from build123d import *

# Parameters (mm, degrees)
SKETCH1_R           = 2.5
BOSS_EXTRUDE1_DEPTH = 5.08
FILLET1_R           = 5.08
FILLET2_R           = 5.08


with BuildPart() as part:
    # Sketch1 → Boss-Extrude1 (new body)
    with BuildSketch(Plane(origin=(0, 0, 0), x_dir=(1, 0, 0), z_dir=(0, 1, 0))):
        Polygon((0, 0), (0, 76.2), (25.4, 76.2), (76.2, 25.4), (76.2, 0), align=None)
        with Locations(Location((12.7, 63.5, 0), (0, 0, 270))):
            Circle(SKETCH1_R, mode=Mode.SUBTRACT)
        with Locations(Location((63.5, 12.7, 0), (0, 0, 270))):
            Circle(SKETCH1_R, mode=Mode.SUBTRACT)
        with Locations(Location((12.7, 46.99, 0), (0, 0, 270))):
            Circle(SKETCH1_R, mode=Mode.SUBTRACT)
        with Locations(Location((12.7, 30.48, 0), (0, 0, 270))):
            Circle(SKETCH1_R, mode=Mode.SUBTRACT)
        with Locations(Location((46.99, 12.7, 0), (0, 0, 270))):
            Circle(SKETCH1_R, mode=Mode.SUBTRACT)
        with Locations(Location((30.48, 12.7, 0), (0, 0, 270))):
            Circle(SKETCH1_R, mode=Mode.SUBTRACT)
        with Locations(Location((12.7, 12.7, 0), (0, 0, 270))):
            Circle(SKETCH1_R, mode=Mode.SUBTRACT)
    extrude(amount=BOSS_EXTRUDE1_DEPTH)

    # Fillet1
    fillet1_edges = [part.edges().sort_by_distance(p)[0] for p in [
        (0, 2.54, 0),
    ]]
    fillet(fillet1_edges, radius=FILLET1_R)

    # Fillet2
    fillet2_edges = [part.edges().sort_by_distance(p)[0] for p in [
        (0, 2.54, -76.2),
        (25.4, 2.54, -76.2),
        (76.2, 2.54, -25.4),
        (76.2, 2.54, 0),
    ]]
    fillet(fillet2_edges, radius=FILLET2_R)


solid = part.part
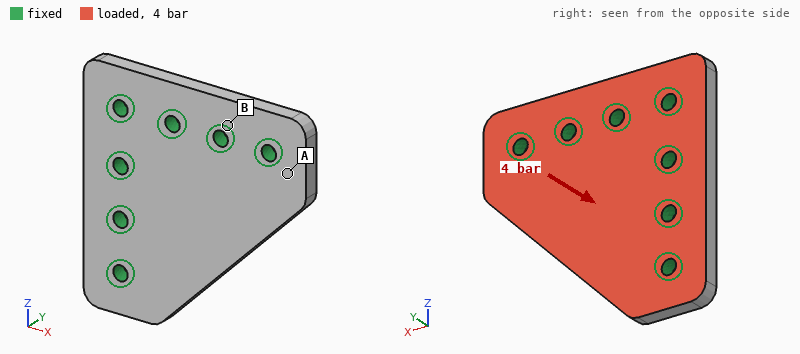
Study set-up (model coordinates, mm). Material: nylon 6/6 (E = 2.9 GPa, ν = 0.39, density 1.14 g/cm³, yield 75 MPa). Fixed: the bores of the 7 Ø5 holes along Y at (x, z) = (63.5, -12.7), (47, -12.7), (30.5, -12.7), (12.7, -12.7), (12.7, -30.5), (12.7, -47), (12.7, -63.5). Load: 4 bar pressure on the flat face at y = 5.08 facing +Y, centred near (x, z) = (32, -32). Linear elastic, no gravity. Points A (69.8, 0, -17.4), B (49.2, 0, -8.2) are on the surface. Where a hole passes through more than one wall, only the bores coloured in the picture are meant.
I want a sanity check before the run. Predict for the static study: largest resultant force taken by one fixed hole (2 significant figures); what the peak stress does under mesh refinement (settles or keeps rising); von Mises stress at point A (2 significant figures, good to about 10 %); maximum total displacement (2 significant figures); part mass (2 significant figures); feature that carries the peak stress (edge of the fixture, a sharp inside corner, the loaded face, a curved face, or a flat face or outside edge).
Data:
330 N
keeps rising
14 MPa
0.92 mm
25 g
edge of the fixture
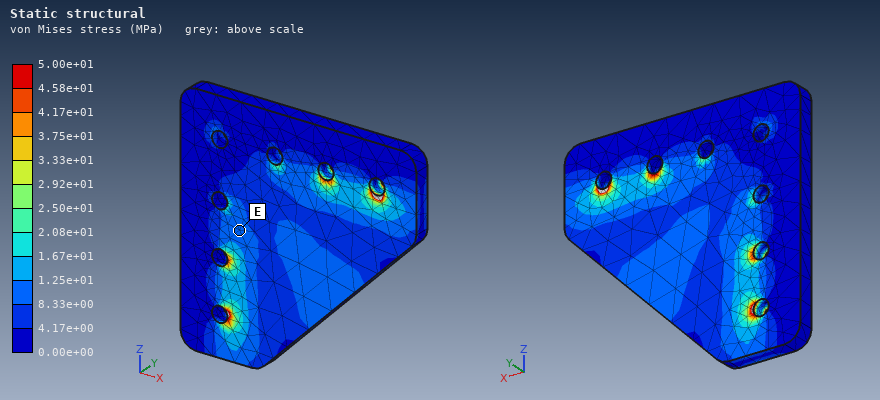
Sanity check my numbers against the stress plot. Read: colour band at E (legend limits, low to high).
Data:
8.33e+00 to 1.25e+01 MPa
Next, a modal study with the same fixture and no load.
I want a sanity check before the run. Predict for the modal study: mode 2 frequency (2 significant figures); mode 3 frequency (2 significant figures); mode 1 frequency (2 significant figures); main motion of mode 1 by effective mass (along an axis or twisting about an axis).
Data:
3700 Hz
5100 Hz
1900 Hz
along Y
